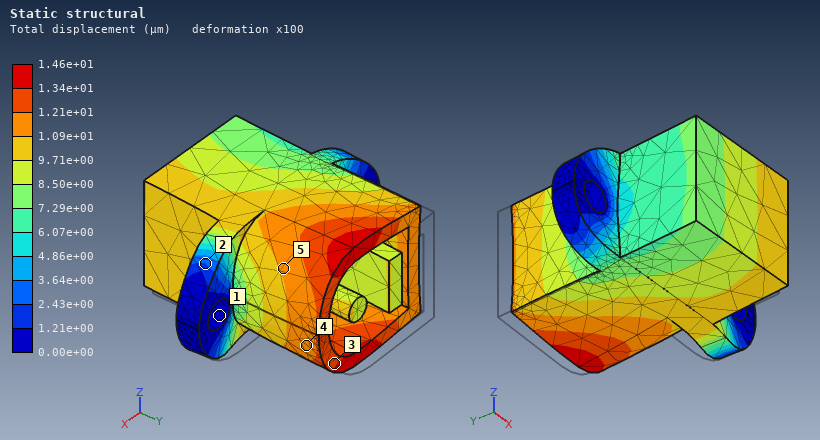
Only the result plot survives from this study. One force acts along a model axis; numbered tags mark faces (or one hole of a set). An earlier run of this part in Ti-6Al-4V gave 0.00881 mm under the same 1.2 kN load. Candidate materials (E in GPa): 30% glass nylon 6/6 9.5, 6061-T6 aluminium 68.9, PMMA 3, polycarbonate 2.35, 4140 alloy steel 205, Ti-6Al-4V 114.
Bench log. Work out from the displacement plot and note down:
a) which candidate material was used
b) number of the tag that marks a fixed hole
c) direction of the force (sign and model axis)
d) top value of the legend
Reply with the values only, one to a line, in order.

6061-T6 aluminium
1
-Y
1.46e+01 µm
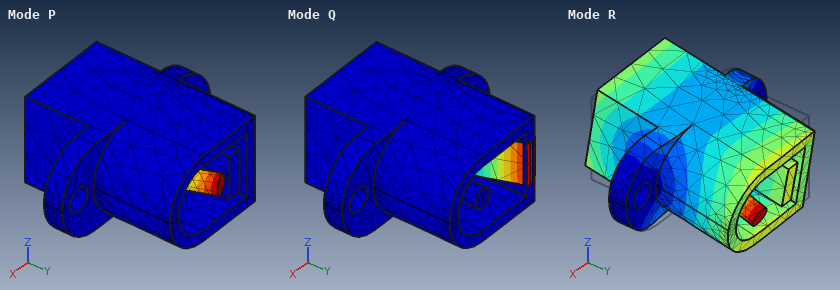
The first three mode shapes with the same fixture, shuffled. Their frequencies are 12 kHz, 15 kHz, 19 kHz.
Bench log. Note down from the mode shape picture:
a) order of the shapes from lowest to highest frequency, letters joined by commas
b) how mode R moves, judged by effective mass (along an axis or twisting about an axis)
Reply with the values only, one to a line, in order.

R, Q, P
twisting about X
